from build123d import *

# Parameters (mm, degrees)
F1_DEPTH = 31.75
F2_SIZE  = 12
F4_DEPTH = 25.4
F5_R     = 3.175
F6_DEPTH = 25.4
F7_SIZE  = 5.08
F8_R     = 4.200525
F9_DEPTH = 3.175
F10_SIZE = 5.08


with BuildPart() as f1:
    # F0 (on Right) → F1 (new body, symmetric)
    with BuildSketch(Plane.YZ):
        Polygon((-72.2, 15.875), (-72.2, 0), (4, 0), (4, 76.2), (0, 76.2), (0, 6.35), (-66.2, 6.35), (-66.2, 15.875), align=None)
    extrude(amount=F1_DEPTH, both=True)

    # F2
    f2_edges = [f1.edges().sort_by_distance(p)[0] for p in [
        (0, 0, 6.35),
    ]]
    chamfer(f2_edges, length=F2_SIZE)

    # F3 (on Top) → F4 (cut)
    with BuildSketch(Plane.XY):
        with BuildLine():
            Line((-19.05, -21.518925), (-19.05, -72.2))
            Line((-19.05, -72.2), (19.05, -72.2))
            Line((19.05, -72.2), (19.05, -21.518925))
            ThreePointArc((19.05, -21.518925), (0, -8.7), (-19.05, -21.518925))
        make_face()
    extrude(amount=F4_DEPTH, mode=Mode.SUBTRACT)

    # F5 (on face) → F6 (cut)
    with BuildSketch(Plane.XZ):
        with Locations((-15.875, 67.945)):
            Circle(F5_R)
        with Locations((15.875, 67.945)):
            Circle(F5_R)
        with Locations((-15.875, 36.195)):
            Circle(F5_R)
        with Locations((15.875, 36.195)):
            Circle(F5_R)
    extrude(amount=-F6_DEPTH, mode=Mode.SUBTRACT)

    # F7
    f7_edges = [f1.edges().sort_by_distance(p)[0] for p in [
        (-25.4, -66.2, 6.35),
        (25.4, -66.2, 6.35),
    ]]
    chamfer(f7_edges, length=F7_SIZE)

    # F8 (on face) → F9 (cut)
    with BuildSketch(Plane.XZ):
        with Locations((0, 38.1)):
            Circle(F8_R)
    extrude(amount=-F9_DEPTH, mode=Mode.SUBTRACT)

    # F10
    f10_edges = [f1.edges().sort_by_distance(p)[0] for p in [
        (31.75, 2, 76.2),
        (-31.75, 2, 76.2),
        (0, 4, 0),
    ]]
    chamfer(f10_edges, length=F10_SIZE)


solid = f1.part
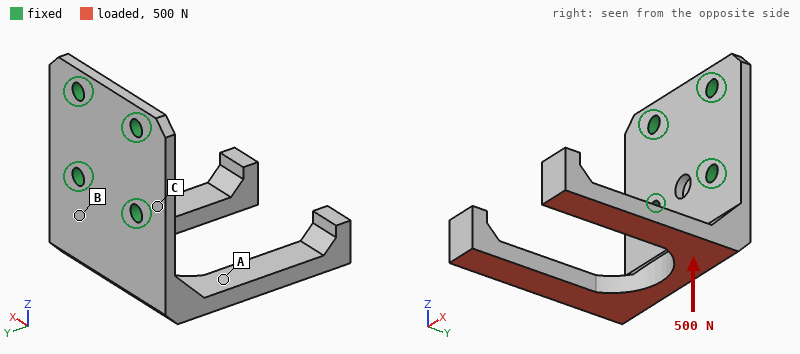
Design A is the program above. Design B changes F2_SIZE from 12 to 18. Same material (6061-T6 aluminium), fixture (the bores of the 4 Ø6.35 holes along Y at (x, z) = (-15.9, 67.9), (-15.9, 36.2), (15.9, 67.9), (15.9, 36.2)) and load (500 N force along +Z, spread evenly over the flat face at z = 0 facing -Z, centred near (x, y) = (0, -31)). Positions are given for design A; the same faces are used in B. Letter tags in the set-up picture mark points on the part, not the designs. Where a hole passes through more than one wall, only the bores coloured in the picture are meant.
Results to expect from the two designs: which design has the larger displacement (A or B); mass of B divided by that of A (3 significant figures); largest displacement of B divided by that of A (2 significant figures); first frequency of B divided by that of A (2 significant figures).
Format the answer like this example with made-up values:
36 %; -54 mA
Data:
A; 1.13; 0.73; 1.1
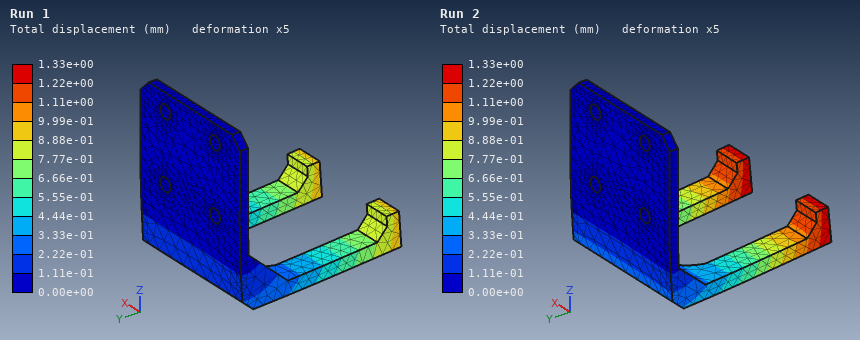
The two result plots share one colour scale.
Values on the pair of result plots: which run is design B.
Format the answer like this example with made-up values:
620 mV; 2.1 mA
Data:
Run 1
